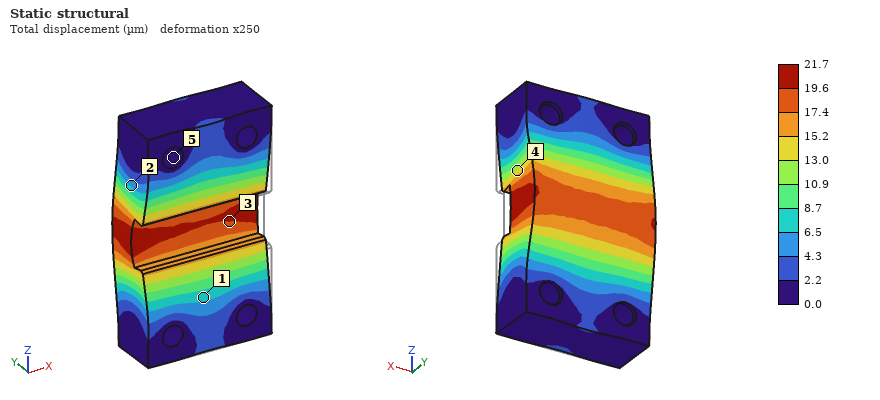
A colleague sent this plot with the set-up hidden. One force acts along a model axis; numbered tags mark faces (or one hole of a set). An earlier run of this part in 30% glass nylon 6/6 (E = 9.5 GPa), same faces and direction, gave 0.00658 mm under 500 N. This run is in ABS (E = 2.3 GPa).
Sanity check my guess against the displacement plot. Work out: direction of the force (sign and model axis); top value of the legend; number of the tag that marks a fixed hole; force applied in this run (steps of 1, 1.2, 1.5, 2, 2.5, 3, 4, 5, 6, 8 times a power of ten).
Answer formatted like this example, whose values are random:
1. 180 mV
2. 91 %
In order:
1. +Y
2. 21.7 µm
3. 5
4. 400 N
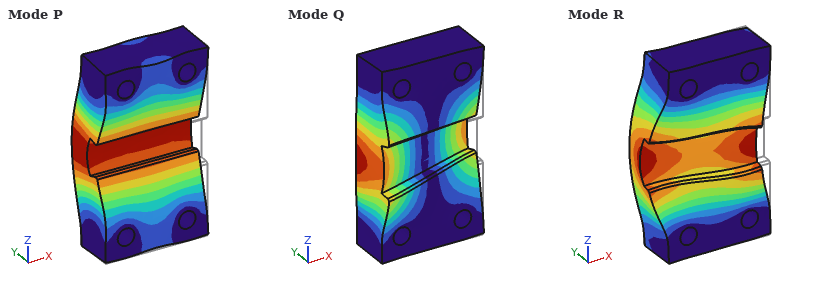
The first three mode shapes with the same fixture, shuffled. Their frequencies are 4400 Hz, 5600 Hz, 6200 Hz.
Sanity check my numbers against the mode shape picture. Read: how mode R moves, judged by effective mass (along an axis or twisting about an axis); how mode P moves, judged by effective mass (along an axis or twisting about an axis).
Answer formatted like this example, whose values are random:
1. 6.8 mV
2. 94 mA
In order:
1. along X
2. along Y
